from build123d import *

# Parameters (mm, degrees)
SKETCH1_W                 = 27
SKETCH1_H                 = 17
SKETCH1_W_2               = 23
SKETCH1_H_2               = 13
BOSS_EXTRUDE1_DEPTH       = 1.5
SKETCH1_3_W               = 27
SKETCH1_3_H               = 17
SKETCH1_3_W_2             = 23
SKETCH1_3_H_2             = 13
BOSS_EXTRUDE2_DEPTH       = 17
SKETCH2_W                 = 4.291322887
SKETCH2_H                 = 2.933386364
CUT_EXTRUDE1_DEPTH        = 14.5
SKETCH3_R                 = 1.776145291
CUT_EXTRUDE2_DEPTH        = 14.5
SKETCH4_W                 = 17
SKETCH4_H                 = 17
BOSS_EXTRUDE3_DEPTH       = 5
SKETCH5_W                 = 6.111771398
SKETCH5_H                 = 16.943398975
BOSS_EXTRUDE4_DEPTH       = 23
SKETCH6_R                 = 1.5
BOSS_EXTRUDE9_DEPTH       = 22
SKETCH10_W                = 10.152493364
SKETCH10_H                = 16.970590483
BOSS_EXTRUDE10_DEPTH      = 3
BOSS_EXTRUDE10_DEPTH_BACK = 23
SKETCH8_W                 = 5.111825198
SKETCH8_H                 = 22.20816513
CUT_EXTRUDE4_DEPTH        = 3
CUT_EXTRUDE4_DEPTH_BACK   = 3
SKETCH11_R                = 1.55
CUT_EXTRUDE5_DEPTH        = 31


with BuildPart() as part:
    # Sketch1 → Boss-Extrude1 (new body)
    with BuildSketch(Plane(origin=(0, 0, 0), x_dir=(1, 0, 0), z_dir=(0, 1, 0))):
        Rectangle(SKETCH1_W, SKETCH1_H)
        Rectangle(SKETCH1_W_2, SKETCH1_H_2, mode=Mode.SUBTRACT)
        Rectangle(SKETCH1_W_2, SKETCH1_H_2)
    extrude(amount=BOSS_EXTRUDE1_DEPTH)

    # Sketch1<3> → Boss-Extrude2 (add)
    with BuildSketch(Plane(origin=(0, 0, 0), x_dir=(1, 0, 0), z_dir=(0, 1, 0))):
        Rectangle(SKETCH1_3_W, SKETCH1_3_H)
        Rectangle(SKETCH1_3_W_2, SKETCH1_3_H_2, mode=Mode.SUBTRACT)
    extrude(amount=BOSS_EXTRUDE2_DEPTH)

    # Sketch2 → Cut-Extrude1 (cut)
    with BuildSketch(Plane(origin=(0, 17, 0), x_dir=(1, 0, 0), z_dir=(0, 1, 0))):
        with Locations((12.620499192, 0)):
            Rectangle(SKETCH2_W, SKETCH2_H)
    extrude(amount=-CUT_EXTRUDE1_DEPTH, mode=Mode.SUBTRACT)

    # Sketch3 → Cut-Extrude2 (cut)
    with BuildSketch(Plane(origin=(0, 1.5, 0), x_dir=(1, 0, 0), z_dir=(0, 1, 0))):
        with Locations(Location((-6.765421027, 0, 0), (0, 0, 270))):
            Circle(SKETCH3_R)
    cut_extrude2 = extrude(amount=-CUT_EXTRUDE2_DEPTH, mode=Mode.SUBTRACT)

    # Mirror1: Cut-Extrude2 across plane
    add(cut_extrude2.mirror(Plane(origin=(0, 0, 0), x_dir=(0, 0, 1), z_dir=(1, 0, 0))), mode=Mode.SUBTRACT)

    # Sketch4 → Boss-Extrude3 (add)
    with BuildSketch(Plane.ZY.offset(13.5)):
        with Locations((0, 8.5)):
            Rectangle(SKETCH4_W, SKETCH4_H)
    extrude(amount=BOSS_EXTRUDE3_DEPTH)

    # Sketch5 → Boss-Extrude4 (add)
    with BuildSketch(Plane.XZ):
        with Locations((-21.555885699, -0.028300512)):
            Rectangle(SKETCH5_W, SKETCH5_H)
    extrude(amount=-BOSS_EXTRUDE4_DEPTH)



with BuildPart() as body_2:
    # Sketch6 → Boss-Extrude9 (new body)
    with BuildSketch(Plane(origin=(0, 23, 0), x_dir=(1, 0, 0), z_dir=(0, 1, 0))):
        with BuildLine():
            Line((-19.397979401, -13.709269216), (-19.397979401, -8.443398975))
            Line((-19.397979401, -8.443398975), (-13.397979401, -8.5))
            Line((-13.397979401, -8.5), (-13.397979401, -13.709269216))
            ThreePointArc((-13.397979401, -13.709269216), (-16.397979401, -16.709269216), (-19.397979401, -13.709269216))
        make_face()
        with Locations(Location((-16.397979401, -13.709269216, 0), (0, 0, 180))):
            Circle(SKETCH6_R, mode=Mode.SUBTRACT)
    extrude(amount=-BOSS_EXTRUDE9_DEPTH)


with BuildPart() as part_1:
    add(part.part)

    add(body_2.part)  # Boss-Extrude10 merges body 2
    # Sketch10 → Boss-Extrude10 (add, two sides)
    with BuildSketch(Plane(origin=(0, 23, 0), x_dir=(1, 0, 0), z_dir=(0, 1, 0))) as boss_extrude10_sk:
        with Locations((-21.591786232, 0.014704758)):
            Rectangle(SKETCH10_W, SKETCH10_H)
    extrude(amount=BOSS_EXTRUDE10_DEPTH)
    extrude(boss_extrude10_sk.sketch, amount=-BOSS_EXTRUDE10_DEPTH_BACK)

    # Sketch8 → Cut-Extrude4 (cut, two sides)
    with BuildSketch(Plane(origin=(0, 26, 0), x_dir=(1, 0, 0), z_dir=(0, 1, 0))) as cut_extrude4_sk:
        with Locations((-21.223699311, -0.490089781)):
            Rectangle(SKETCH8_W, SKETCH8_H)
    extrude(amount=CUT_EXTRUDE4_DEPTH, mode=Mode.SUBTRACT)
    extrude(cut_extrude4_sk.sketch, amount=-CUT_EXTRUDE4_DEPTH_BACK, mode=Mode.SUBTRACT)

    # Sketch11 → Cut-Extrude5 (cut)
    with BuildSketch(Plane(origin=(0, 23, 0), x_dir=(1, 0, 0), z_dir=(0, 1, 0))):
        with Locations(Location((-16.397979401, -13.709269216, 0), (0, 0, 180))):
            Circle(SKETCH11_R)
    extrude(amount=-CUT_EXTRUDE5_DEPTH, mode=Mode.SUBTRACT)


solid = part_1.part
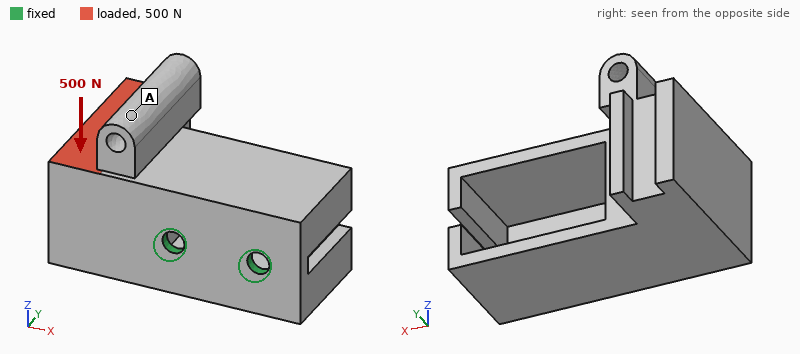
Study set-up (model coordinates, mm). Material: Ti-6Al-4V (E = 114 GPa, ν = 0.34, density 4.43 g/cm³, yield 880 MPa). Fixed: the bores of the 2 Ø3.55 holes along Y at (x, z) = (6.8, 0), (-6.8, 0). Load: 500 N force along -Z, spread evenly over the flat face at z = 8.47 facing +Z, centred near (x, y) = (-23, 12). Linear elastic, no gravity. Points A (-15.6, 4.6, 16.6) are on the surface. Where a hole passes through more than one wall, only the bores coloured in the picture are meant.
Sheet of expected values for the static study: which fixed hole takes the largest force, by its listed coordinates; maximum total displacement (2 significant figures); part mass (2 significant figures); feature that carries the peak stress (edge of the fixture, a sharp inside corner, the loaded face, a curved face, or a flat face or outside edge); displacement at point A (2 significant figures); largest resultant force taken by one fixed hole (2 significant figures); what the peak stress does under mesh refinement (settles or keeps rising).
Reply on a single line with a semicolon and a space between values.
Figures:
(-6.8, 0); 0.16 mm; 40 g; edge of the fixture; 0.098 mm; 930 N; keeps rising
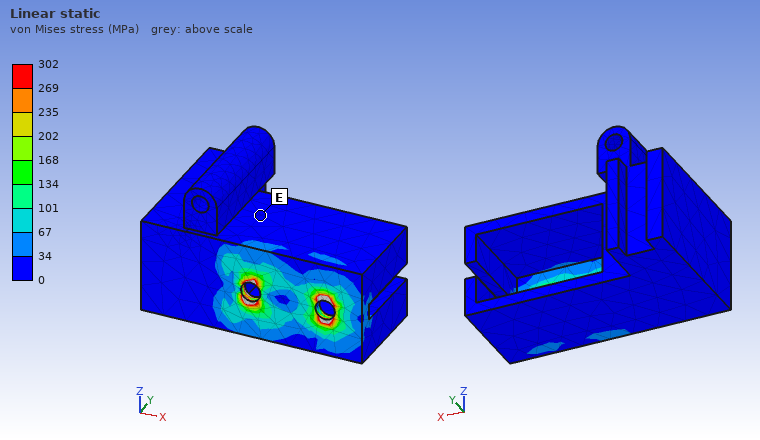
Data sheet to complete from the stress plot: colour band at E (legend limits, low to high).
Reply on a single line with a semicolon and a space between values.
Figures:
0 to 34 MPa
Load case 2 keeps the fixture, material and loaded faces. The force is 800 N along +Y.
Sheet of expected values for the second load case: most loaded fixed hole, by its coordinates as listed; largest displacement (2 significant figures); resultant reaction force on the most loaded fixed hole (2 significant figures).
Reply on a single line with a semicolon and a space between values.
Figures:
(-6.8, 0); 0.26 mm; 1.5 kN
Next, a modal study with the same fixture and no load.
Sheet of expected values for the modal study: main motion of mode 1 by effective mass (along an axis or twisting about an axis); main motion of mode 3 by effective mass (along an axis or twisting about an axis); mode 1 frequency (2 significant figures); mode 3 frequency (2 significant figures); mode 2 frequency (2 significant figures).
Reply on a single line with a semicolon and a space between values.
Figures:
along Z; along Y; 1900 Hz; 6600 Hz; 2700 Hz
